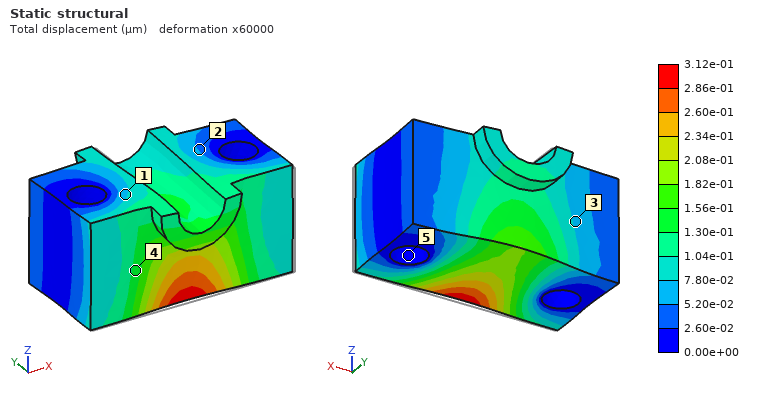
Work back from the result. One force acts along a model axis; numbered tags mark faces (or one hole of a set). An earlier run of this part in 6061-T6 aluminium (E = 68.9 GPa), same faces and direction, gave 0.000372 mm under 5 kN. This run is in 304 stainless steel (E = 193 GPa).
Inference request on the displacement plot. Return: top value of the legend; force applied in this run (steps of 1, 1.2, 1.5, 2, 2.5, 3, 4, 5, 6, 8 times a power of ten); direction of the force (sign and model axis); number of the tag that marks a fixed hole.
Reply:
3.12e-01 µm
12 kN
+Y
5
